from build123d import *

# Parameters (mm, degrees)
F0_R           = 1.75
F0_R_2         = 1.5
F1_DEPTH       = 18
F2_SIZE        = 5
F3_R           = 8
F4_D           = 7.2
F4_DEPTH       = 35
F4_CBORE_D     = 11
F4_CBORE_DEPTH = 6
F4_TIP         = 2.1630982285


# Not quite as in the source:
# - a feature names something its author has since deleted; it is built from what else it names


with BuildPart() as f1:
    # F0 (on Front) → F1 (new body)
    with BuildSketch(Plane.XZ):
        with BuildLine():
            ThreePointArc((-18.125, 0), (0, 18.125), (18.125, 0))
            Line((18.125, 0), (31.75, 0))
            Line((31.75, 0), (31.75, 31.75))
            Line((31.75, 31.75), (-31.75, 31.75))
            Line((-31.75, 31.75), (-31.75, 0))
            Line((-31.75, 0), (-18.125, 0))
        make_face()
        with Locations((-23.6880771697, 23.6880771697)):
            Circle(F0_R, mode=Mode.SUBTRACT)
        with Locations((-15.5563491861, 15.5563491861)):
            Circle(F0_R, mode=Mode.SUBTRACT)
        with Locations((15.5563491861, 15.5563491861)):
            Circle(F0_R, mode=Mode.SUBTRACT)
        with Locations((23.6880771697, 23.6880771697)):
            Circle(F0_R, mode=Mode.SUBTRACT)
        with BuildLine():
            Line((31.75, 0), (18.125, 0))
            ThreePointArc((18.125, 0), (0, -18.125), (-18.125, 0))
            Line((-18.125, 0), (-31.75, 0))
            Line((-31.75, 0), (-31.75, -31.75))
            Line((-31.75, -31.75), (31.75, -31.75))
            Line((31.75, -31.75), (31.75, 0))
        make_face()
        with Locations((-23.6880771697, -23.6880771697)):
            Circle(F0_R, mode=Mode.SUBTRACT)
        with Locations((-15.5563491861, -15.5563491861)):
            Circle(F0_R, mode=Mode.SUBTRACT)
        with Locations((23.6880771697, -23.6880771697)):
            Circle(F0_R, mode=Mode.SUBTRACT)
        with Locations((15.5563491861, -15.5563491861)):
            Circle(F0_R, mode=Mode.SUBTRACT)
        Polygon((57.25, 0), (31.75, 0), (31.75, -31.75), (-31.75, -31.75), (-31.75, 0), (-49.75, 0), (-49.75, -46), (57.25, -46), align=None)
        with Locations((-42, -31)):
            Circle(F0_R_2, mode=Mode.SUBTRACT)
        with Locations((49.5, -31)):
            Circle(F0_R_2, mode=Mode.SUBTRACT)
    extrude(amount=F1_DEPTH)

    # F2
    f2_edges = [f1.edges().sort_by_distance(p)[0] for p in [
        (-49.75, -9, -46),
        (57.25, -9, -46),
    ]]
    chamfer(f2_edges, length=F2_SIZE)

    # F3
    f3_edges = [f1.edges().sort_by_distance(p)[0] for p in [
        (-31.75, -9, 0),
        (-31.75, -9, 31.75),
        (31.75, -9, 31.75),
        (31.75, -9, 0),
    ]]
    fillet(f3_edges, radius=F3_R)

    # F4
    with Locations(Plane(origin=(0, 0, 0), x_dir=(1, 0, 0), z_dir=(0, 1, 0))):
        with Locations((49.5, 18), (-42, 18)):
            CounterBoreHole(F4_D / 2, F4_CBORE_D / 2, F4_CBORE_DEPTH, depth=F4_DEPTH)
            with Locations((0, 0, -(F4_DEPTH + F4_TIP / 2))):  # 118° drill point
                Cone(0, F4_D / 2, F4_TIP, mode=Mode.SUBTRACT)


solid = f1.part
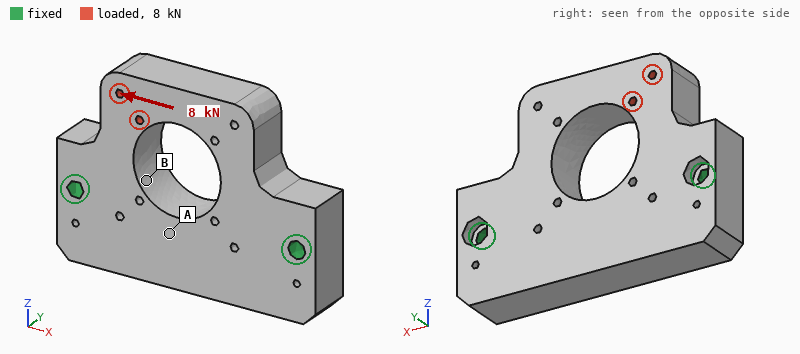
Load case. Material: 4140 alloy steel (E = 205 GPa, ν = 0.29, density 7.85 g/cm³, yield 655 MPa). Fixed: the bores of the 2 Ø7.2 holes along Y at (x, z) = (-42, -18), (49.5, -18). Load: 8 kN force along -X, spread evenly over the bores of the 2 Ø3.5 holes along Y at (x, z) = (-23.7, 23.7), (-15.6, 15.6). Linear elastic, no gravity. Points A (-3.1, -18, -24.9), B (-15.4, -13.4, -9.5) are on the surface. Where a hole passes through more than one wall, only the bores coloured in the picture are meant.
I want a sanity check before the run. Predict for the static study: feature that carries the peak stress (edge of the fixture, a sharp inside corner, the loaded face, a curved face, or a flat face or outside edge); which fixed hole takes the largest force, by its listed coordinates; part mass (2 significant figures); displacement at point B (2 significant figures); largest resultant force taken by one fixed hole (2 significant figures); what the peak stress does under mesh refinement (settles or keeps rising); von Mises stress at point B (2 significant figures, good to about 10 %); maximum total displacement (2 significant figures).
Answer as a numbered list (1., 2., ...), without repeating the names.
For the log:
1. edge of the fixture
2. (-42, -18)
3. 800 g
4. 3.2 µm
5. 5.9 kN
6. keeps rising
7. 34 MPa
8. 14 µm
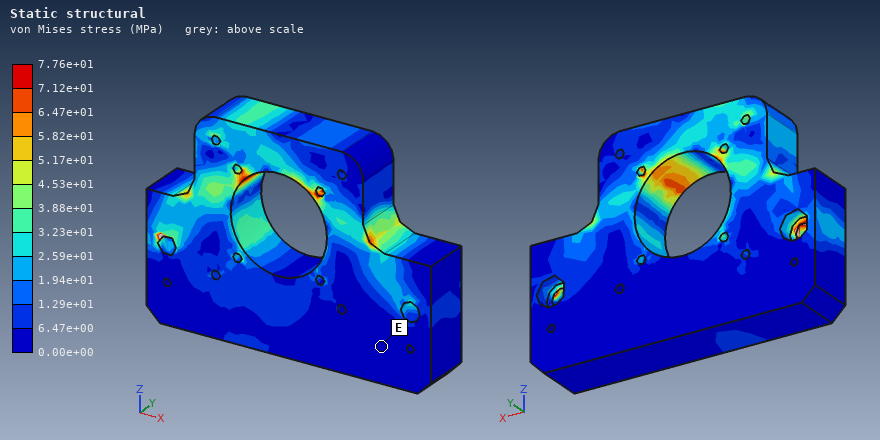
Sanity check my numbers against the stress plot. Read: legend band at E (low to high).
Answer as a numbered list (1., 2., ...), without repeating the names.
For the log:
1. 0.00e+00 to 6.47e+00 MPa
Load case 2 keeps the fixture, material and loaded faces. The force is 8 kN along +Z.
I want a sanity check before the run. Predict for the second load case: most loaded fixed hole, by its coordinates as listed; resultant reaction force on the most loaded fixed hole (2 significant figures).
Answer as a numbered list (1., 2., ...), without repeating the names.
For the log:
1. (-42, -18)
2. 6.1 kN
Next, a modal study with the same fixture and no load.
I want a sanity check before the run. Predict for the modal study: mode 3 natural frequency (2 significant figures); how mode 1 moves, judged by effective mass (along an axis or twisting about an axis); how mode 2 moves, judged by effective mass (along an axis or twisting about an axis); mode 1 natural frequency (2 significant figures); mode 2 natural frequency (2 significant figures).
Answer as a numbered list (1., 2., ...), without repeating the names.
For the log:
1. 8000 Hz
2. along Y
3. along Y
4. 3300 Hz
5. 5900 Hz
